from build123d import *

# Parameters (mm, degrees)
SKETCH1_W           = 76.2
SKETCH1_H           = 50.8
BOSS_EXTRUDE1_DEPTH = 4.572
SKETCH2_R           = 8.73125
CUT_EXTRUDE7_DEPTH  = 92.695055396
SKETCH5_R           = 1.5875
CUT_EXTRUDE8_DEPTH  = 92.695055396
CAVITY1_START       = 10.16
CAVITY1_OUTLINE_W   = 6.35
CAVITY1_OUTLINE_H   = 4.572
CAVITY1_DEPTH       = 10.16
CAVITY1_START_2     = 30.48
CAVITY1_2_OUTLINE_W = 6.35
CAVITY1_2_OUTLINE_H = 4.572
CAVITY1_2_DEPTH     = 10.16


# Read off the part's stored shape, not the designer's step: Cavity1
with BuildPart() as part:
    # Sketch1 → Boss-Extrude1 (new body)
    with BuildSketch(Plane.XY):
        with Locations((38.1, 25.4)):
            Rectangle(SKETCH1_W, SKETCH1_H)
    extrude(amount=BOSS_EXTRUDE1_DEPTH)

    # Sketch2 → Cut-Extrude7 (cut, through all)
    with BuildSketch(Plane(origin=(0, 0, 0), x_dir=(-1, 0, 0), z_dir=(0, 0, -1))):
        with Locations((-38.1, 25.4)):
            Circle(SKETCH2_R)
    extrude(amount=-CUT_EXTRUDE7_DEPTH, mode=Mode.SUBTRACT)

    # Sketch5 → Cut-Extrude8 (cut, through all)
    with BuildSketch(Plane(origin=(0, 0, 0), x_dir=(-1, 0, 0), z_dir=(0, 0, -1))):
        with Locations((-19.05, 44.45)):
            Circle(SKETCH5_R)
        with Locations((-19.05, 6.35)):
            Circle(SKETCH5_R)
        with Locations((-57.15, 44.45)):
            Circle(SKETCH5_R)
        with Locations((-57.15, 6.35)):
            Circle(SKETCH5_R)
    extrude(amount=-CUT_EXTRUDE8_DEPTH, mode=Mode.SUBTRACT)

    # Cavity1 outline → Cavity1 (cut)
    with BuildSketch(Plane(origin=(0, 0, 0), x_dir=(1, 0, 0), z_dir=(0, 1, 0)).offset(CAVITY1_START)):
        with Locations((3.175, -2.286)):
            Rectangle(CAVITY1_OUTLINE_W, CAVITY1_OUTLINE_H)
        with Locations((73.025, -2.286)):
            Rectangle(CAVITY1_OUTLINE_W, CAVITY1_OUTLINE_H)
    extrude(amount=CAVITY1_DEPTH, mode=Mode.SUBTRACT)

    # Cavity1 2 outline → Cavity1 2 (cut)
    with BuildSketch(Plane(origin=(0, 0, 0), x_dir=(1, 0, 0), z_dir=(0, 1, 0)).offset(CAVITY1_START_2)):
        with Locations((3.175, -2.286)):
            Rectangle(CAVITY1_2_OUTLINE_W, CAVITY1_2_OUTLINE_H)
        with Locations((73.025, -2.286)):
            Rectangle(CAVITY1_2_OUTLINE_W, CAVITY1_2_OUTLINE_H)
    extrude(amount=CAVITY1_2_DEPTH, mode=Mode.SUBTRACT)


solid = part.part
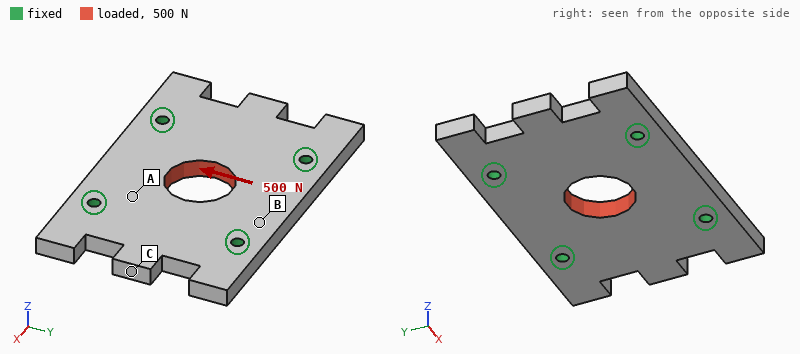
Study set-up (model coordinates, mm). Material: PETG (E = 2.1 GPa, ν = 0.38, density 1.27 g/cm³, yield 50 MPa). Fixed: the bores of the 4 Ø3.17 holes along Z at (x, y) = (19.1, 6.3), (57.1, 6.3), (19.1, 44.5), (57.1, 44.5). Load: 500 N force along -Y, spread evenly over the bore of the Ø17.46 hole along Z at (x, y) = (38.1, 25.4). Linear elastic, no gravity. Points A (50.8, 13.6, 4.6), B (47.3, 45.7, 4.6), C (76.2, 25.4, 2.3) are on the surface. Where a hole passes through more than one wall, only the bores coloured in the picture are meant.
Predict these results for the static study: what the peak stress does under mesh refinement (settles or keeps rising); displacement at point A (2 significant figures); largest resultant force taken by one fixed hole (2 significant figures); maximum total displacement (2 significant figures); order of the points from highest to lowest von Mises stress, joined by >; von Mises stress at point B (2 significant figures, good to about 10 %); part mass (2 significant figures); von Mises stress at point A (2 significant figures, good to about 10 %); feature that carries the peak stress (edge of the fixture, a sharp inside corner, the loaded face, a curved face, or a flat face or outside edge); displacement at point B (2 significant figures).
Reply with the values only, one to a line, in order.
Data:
keeps rising
15 µm
140 N
33 µm
A > B > C
1.3 MPa
19 g
2.3 MPa
edge of the fixture
19 µm
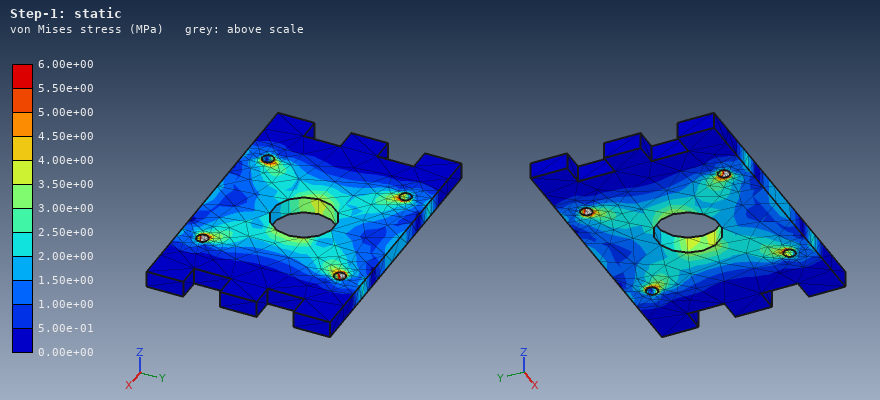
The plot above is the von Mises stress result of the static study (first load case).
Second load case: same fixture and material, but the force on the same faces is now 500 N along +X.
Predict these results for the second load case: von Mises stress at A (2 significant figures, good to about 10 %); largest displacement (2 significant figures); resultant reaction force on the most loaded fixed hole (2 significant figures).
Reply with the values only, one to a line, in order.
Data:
2.0 MPa
28 µm
130 N
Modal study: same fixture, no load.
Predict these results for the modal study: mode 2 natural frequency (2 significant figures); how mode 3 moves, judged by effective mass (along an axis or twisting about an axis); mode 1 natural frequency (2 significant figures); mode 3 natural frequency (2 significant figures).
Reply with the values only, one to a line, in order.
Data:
2300 Hz
along Z
2200 Hz
2900 Hz
